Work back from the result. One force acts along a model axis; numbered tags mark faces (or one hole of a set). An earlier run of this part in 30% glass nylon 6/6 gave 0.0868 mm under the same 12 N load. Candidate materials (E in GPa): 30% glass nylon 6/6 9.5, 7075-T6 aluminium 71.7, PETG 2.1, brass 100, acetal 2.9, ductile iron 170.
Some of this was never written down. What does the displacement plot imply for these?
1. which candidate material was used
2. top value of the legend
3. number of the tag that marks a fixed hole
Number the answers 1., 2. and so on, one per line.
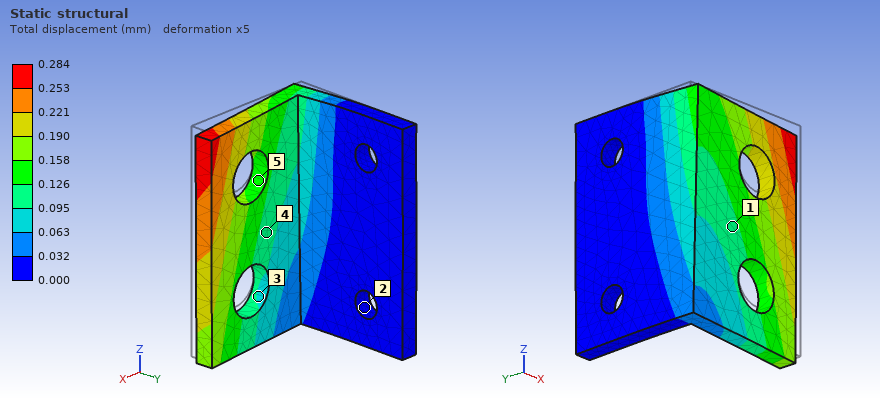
1. acetal
2. 0.284 mm
3. 2
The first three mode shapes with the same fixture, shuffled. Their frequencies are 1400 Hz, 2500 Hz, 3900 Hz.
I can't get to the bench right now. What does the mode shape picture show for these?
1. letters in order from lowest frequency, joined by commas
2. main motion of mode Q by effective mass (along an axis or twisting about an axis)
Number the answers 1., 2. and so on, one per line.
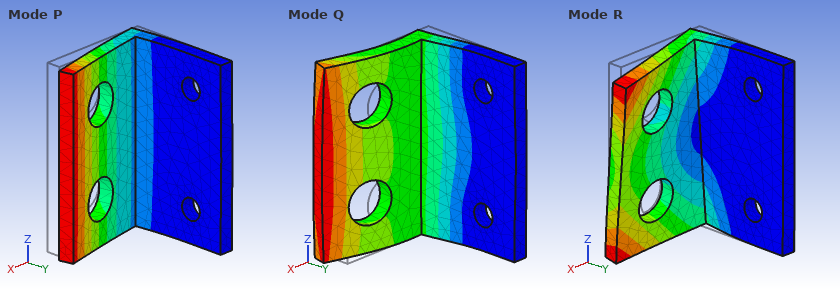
1. P, R, Q
2. along X
